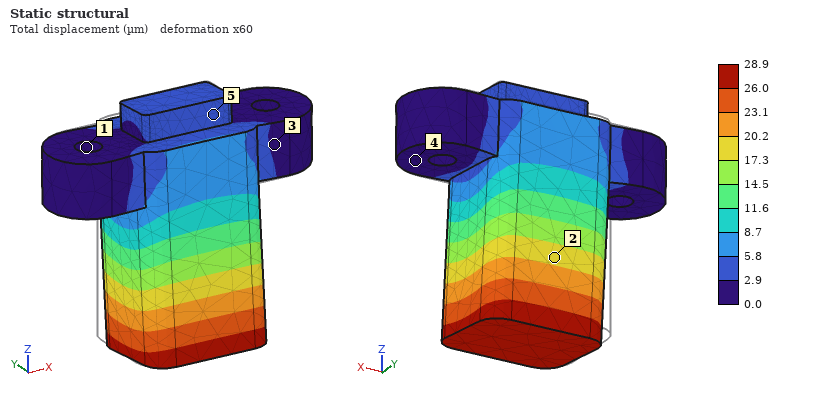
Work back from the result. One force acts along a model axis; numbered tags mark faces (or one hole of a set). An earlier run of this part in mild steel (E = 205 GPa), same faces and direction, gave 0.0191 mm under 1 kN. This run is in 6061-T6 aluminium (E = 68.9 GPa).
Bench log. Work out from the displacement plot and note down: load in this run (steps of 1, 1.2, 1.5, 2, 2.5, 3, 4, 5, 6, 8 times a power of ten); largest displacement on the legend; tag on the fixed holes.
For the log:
500 N
28.9 µm
1
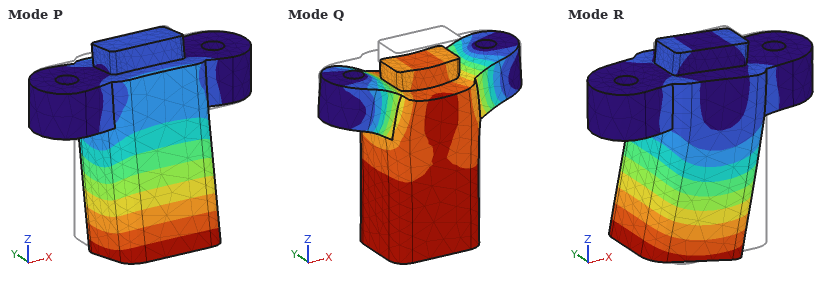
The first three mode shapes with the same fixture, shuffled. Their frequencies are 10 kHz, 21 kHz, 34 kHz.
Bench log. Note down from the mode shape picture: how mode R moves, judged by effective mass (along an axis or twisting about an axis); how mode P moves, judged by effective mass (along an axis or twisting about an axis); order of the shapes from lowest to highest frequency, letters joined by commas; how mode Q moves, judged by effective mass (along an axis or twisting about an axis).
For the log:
along X
along Y
P, R, Q
along Z
